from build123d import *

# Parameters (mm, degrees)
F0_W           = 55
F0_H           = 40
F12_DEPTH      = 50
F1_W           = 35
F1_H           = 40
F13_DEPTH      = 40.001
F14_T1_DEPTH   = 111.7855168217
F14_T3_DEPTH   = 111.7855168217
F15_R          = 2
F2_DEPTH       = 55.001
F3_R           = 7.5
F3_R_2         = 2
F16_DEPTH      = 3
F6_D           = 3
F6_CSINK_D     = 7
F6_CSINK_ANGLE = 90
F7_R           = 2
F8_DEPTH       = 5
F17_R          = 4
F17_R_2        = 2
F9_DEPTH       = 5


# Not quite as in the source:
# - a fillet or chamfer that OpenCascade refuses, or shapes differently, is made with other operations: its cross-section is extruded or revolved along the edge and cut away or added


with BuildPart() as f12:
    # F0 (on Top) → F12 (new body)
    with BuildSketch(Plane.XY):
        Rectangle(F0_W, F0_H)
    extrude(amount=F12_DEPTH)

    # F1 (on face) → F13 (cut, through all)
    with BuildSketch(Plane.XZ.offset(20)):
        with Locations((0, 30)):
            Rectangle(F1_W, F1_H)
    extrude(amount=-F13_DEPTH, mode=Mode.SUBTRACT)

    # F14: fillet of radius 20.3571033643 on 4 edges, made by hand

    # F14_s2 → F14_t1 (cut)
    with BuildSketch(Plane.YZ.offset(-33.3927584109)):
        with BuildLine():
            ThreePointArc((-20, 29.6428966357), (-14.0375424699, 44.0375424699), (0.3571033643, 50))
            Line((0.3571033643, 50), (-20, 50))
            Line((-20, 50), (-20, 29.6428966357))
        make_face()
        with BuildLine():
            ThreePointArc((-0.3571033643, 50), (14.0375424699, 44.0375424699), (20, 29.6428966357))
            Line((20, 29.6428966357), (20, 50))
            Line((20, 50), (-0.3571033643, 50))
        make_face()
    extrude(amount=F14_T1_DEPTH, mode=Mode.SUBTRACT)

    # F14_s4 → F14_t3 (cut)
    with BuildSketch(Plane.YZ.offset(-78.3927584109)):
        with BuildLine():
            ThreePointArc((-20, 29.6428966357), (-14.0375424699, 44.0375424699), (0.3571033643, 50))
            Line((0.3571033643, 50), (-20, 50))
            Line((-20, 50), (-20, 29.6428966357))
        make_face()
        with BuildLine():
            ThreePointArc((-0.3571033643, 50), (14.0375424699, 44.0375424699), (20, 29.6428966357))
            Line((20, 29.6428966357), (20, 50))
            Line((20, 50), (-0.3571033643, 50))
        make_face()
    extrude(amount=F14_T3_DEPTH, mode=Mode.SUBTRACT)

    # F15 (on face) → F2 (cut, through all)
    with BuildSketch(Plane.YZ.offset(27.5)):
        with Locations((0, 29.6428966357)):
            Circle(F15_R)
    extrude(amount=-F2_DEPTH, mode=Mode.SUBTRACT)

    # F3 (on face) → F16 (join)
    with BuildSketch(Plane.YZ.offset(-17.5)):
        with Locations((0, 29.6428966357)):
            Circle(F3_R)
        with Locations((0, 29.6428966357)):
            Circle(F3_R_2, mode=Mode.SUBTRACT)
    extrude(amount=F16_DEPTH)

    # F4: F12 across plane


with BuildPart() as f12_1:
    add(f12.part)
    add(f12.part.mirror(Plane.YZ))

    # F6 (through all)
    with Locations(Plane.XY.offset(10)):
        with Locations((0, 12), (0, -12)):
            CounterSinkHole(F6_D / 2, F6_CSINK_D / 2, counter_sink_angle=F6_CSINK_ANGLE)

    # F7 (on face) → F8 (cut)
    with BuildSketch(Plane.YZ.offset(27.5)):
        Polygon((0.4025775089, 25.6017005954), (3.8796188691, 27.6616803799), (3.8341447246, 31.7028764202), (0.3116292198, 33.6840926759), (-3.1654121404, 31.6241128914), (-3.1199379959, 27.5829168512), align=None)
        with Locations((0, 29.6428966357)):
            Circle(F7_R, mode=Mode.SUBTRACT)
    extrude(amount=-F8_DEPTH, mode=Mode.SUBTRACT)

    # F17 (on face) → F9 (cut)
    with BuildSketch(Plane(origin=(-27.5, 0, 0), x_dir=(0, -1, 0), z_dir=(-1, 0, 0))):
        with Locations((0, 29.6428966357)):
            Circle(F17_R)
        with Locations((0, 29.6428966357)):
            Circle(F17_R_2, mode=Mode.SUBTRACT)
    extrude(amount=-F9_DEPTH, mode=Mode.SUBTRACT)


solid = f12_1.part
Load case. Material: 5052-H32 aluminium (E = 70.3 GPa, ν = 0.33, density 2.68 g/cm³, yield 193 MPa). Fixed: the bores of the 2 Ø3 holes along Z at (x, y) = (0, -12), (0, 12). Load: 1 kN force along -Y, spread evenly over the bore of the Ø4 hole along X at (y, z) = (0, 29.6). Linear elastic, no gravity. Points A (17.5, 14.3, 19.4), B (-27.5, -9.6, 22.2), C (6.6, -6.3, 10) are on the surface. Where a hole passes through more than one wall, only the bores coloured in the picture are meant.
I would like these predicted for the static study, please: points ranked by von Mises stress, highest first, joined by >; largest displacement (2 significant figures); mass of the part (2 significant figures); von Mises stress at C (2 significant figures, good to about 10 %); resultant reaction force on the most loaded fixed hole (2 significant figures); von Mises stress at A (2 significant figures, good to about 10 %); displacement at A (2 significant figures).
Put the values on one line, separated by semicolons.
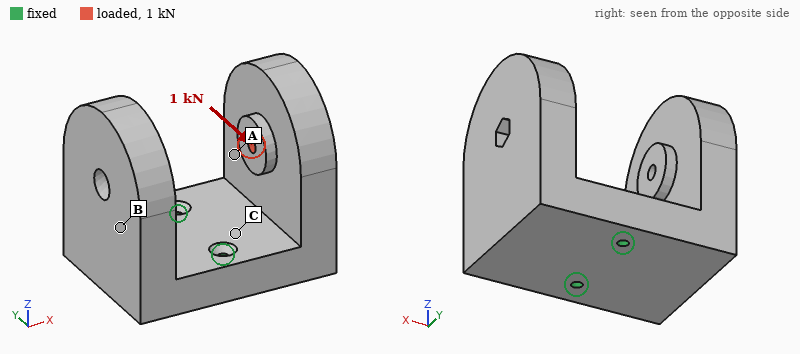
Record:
C > A > B; 57 µm; 140 g; 26 MPa; 1.2 kN; 12 MPa; 26 µm
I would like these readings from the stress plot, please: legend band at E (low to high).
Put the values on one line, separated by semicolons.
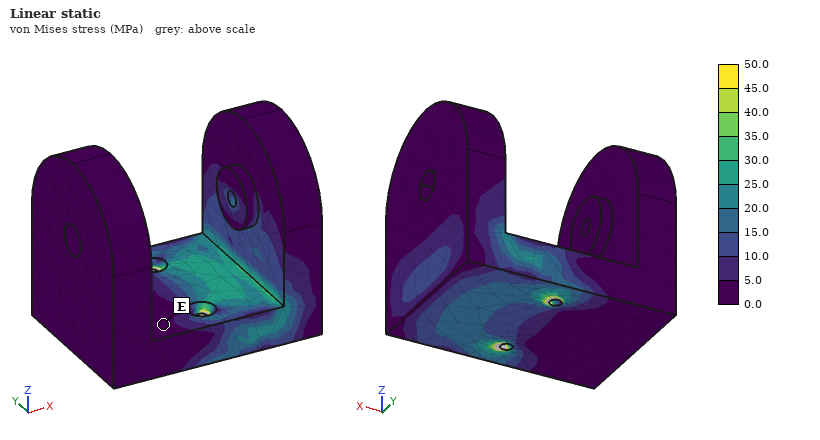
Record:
0.0 to 5.0 MPa
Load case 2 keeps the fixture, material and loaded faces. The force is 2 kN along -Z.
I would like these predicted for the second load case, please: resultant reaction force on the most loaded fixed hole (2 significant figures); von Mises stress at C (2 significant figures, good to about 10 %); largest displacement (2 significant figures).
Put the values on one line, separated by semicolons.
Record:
1.0 kN; 29 MPa; 0.11 mm
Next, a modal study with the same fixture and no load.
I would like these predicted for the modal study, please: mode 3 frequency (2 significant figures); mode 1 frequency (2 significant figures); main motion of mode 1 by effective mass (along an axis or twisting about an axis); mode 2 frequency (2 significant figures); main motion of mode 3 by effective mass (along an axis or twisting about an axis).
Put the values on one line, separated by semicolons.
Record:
4000 Hz; 2000 Hz; along X; 2600 Hz; twisting about Z
